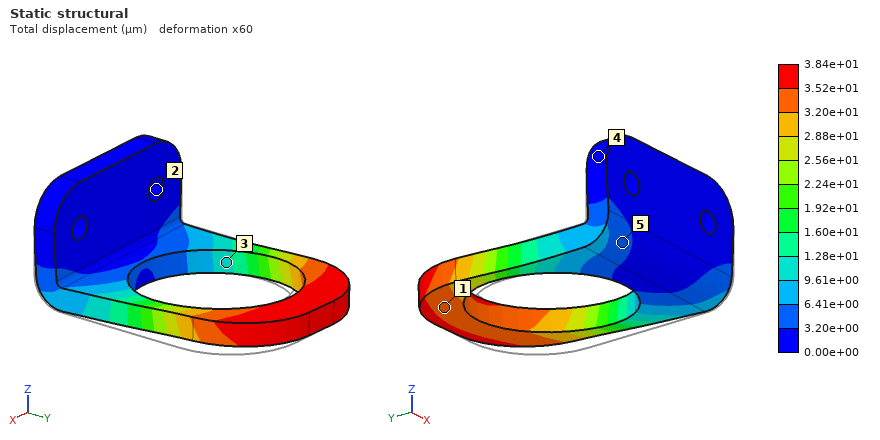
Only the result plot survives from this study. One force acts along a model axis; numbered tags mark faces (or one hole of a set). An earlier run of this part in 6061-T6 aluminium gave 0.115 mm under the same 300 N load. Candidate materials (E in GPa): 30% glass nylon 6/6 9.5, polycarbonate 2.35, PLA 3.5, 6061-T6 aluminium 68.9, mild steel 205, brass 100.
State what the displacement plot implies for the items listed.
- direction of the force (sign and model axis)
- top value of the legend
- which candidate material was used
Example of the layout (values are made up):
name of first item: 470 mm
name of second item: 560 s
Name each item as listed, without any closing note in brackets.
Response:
direction of the force: -X
top value of the legend: 3.84e+01 µm
which candidate material was used: mild steel
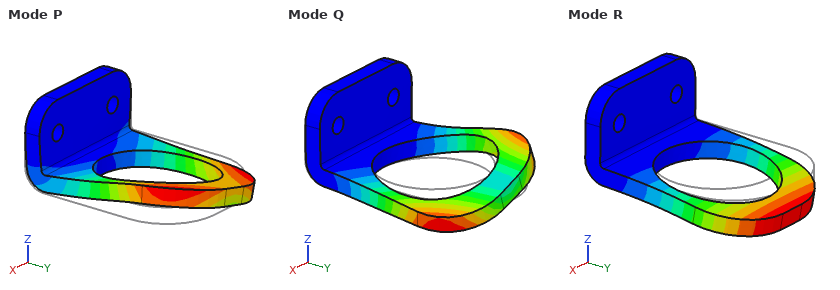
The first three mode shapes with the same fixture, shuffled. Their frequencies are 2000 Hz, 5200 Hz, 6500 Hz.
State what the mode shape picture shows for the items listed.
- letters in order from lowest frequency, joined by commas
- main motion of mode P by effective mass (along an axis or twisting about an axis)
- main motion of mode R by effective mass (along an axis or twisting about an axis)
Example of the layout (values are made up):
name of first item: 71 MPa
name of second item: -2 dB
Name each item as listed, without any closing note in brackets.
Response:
letters in order from lowest frequency, joined by commas: R, P, Q
main motion of mode P by effective mass: along X
main motion of mode R by effective mass: along Z
